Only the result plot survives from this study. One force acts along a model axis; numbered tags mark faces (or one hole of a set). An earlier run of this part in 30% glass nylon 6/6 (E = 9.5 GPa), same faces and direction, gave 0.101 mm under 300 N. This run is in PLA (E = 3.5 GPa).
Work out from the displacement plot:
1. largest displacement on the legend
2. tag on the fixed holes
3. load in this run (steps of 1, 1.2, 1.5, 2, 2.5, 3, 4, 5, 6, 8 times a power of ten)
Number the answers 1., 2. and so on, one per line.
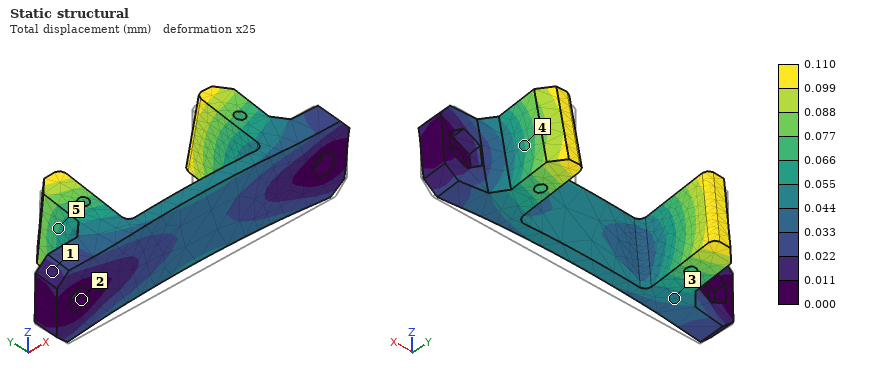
1. 0.110 mm
2. 2
3. 120 N
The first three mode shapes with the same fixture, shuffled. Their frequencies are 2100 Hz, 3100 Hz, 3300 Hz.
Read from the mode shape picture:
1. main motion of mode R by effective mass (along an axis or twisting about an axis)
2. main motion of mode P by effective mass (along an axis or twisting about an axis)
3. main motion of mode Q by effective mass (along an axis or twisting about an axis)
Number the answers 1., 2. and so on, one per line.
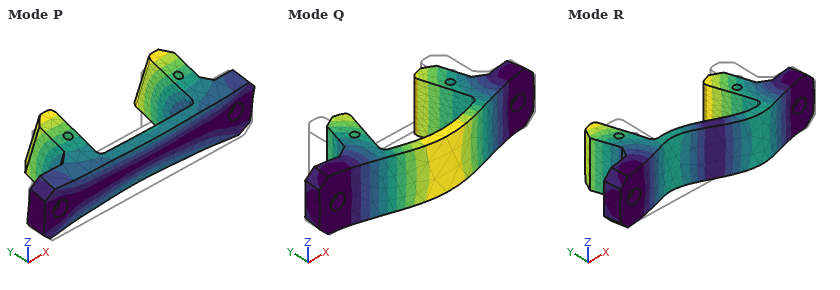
1. along X
2. along Z
3. along Y
